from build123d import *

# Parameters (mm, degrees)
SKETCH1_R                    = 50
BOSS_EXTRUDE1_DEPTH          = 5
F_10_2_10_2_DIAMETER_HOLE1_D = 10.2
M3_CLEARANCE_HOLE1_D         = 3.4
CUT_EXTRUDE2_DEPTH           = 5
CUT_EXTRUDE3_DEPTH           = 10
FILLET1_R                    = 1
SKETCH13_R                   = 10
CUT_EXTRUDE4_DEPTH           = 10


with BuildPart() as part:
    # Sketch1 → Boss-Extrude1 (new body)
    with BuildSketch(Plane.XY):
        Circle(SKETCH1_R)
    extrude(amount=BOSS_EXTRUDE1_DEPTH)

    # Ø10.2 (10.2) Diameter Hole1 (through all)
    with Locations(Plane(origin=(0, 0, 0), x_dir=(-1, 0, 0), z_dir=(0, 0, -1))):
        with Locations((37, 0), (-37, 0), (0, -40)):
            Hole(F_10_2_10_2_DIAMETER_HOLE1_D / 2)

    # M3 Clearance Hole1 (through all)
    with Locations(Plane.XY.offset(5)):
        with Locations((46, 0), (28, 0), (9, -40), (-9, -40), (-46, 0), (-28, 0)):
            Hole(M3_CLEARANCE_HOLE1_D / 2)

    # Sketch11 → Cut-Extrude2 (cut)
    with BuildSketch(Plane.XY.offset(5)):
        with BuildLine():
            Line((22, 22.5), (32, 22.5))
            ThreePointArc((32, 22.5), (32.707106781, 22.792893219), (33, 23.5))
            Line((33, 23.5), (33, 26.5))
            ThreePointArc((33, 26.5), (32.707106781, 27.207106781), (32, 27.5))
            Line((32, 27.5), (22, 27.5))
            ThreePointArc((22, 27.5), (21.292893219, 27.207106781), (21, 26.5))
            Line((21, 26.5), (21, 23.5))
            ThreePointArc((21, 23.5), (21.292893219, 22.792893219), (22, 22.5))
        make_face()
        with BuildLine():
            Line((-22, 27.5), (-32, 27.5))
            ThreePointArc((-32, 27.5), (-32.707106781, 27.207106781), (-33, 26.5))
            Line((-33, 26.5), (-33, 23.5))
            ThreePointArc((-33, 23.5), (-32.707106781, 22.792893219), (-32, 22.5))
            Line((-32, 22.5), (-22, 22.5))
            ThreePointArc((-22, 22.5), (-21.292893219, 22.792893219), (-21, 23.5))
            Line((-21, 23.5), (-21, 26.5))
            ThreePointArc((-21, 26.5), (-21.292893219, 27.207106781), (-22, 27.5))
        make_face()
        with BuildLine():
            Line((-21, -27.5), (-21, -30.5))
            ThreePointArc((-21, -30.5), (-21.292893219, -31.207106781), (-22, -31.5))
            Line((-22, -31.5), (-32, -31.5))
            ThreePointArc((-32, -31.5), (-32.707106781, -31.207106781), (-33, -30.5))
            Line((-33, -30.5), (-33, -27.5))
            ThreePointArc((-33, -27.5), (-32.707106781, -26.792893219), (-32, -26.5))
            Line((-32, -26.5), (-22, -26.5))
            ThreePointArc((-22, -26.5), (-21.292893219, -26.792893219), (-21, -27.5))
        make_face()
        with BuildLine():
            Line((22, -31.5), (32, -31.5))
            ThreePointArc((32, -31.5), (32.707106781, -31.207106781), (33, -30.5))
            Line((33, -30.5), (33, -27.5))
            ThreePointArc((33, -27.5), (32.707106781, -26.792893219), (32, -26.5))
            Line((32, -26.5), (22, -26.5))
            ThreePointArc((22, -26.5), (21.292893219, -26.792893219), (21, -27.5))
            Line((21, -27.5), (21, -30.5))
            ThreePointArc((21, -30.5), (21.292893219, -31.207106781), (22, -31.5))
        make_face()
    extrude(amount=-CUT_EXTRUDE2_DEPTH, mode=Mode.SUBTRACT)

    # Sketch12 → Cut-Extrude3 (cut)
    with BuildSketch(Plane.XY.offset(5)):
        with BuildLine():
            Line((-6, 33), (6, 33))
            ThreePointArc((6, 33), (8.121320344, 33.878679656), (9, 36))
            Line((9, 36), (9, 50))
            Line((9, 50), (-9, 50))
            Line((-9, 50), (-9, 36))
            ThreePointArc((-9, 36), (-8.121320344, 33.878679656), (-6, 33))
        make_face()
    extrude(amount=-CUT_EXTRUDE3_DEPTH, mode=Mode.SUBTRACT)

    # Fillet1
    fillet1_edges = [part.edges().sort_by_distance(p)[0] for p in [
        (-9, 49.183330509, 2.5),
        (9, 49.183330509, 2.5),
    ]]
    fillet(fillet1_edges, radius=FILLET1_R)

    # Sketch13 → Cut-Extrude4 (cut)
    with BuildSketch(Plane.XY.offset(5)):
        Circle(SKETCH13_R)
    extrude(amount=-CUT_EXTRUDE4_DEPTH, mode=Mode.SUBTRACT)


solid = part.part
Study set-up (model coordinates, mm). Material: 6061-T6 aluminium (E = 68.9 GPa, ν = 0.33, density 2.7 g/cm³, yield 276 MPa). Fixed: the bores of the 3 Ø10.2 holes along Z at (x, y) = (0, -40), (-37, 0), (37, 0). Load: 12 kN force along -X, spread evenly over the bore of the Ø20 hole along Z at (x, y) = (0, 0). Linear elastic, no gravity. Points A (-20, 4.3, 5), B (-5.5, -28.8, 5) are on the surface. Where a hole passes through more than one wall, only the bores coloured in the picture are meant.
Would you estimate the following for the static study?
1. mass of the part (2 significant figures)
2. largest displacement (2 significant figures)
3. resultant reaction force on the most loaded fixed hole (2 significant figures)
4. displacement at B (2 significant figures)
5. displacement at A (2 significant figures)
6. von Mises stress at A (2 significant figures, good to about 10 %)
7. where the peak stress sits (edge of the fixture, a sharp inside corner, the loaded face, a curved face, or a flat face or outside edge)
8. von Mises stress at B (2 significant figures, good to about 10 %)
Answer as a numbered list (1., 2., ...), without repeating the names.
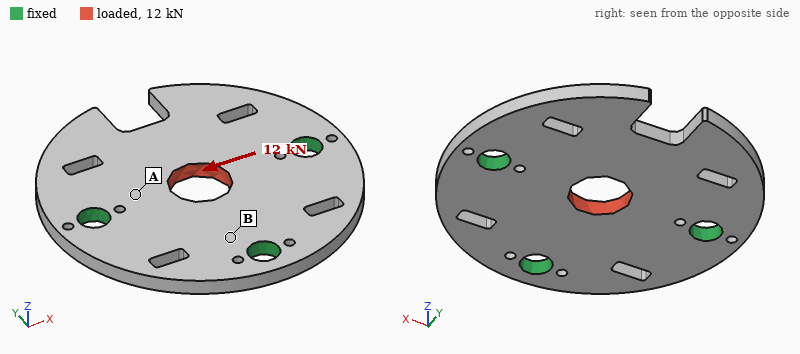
1. 91 g
2. 21 µm
3. 5.2 kN
4. 4.5 µm
5. 11 µm
6. 45 MPa
7. a curved face
8. 11 MPa
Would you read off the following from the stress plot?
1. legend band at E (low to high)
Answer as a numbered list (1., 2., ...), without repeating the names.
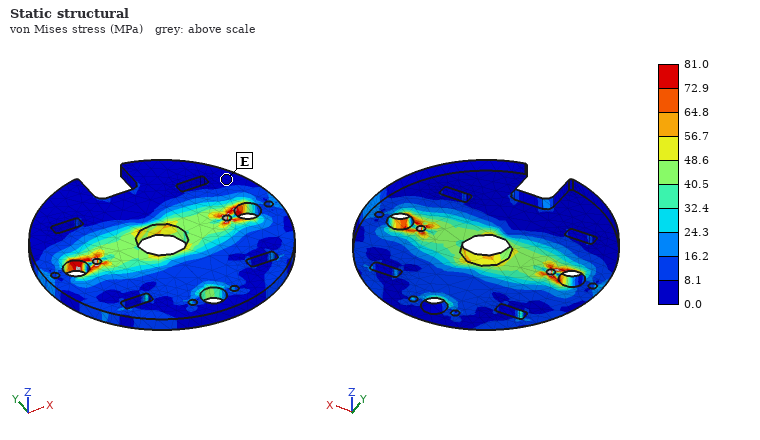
1. 0.0 to 8.1 MPa
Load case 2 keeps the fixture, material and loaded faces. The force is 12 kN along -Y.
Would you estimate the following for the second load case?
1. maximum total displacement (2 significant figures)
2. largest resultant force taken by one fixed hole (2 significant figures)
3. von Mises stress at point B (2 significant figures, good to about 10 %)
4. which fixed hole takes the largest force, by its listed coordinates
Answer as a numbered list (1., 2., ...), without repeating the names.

1. 31 µm
2. 5.1 kN
3. 46 MPa
4. (0, -40)
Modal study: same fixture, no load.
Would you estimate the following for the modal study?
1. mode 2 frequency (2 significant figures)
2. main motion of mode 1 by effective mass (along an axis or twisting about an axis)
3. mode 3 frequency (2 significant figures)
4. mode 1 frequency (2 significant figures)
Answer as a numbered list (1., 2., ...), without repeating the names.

1. 4000 Hz
2. along Z
3. 6400 Hz
4. 2200 Hz
